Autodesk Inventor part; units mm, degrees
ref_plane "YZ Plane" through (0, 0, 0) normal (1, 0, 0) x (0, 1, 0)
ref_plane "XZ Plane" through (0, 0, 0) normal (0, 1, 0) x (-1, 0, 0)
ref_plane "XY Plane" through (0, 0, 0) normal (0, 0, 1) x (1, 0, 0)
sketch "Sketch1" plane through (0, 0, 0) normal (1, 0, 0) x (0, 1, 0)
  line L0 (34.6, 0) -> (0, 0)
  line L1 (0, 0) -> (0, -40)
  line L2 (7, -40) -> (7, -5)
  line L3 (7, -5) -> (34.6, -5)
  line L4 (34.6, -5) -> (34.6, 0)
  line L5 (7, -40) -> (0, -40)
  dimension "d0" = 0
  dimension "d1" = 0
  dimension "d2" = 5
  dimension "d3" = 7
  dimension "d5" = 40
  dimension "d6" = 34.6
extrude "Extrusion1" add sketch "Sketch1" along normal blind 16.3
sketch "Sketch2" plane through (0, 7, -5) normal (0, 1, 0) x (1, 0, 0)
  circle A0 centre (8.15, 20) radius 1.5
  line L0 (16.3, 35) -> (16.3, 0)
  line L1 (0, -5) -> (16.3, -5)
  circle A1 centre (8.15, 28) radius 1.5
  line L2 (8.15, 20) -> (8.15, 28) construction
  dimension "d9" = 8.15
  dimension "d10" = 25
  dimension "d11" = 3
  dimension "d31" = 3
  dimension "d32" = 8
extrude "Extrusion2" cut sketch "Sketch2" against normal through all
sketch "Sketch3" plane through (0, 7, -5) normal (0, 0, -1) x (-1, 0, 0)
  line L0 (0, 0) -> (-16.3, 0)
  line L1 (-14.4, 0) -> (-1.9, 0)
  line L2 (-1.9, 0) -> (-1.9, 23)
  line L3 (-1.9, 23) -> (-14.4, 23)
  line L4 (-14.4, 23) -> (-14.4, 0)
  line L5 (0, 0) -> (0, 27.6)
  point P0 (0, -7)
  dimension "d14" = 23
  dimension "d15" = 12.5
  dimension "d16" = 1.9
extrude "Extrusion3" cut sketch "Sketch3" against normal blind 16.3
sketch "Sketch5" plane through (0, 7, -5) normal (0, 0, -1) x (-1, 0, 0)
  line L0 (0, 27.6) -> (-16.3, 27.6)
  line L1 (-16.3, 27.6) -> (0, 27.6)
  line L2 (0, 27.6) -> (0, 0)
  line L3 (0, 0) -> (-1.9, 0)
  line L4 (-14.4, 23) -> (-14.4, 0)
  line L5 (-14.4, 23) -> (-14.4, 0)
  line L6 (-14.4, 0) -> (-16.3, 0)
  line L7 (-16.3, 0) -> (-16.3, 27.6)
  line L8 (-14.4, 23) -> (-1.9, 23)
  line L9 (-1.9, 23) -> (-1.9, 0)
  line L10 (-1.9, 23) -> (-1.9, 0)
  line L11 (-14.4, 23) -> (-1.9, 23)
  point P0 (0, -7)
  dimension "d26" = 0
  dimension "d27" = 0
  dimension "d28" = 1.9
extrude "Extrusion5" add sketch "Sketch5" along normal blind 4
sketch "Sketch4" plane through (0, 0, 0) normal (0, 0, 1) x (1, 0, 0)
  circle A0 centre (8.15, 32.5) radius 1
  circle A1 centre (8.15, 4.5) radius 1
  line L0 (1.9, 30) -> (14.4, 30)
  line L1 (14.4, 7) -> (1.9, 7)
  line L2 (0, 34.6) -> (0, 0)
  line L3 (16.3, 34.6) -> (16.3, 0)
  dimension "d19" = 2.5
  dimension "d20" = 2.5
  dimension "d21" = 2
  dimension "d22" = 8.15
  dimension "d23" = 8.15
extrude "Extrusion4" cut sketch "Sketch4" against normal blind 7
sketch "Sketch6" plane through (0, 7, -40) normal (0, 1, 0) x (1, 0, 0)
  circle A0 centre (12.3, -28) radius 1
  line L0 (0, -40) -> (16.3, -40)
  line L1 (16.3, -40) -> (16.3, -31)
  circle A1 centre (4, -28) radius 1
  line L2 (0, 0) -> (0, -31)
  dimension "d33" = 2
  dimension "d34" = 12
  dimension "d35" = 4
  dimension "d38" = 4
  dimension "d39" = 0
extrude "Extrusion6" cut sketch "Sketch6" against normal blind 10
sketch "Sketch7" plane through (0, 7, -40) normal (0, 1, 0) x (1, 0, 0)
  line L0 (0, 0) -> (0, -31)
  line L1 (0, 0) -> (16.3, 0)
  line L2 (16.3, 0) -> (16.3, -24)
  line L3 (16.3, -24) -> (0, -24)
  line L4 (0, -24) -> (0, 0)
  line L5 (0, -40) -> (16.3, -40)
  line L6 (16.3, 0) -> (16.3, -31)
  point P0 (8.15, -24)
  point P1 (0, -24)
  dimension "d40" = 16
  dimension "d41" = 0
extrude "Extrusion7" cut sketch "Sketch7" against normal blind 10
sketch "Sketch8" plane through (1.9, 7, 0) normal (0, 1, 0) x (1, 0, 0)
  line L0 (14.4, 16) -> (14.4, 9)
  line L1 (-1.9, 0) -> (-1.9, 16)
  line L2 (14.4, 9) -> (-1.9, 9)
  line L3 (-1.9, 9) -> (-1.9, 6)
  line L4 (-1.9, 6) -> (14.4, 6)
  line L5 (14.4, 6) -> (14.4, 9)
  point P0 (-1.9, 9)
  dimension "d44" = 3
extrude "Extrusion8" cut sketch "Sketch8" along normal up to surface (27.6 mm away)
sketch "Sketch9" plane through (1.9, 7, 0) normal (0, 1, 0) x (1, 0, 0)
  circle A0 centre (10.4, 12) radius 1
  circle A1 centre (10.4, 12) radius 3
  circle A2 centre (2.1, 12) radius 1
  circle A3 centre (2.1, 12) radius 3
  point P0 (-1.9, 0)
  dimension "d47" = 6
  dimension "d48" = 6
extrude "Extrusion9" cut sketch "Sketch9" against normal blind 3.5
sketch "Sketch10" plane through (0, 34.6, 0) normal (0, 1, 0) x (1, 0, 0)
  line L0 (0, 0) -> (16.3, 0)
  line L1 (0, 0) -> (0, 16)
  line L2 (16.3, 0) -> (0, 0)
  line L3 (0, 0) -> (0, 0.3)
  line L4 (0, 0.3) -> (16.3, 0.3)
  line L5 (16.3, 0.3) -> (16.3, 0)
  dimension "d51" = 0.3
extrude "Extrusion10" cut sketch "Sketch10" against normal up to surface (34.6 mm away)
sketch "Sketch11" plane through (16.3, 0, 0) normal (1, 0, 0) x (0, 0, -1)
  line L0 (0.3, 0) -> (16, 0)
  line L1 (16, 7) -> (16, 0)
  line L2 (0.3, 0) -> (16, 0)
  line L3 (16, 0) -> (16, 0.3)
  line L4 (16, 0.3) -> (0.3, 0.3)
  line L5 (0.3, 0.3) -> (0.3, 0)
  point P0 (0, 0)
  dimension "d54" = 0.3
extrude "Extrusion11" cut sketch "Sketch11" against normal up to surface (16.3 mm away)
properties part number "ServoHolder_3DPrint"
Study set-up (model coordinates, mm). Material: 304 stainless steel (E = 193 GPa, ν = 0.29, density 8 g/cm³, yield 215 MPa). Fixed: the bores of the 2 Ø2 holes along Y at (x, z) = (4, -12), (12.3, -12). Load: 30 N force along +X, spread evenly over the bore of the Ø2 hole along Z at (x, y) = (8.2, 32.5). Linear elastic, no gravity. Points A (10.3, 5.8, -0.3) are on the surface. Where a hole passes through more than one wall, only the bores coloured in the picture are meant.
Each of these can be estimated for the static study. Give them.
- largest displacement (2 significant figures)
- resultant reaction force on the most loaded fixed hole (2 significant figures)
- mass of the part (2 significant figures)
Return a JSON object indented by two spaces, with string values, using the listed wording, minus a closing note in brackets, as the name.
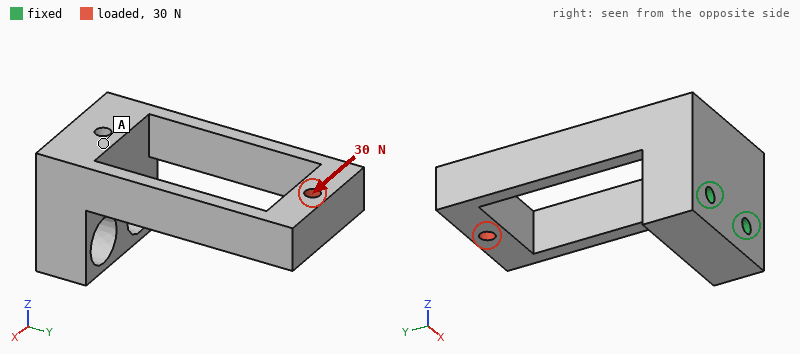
{
  "largest displacement": "36 µm",
  "resultant reaction force on the most loaded fixed hole": "91 N",
  "mass of the part": "19 g"
}
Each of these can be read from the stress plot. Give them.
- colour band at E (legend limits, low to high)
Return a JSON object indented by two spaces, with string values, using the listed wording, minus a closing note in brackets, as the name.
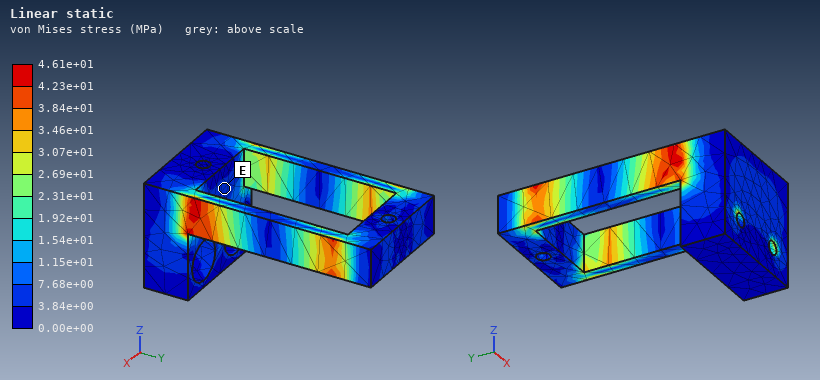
{
  "colour band at E": "3.84e+00 to 7.68e+00 MPa"
}
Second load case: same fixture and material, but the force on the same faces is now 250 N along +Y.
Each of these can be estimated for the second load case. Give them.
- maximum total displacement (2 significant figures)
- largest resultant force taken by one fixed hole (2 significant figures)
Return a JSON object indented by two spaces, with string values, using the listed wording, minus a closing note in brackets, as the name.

{
  "maximum total displacement": "20 µm",
  "largest resultant force taken by one fixed hole": "130 N"
}
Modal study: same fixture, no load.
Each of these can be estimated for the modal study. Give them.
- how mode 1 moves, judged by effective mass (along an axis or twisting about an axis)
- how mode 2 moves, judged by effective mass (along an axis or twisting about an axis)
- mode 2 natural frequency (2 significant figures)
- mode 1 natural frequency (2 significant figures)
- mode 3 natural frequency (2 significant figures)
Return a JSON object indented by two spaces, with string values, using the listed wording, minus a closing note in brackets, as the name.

{
  "how mode 1 moves, judged by effective mass": "along X",
  "how mode 2 moves, judged by effective mass": "along Z",
  "mode 2 natural frequency": "2600 Hz",
  "mode 1 natural frequency": "2200 Hz",
  "mode 3 natural frequency": "6800 Hz"
}
